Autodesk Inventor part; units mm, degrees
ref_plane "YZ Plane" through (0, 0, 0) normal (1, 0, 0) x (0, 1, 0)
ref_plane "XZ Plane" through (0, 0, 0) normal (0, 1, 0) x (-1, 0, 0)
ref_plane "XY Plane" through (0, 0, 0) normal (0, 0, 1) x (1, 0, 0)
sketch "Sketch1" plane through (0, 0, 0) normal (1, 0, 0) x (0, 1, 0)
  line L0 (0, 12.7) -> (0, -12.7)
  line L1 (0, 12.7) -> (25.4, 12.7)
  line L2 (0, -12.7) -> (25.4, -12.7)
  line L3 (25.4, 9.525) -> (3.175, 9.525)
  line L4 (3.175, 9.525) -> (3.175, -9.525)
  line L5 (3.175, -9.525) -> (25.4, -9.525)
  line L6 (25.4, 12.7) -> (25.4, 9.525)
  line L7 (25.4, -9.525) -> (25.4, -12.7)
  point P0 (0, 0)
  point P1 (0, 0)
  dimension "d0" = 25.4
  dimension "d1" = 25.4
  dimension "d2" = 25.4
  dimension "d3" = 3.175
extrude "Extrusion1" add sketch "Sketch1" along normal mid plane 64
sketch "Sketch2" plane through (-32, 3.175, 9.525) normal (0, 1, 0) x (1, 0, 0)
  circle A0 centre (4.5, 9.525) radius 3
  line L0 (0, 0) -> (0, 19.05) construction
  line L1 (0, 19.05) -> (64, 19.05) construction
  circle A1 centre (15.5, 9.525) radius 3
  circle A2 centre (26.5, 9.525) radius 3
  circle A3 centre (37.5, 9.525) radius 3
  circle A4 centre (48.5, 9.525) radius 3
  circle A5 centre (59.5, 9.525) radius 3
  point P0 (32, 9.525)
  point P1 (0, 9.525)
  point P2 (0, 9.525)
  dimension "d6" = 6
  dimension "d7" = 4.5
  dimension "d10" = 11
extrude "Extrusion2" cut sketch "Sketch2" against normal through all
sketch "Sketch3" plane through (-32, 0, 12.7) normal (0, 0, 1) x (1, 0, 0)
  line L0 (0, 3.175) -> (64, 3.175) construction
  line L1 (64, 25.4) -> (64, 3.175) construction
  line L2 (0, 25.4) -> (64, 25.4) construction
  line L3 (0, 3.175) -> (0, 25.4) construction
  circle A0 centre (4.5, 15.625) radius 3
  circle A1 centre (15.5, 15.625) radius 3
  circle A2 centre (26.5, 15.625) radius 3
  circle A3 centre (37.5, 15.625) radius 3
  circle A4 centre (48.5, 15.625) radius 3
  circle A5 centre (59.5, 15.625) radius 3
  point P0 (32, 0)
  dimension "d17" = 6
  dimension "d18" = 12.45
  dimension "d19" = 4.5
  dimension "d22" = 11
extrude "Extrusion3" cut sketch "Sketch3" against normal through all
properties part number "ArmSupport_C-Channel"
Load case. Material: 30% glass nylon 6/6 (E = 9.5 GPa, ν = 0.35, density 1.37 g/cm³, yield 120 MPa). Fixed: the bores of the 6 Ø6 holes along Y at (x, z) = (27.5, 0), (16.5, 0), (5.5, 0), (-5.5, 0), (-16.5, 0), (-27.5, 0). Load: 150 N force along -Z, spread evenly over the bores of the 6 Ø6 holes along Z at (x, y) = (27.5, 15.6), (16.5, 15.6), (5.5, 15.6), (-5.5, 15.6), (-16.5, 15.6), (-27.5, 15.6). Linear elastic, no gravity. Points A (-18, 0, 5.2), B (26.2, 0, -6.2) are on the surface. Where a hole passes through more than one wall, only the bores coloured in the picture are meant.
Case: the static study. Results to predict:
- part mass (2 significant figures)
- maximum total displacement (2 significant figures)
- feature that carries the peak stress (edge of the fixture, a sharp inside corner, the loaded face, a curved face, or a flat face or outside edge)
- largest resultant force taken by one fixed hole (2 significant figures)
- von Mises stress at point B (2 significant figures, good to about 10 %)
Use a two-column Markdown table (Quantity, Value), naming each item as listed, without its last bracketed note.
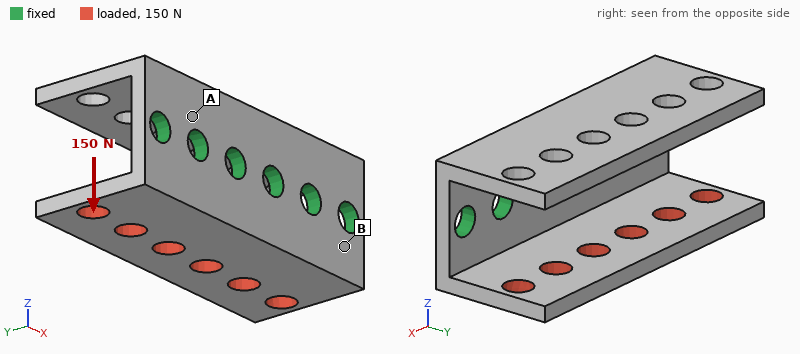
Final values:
| Quantity | Value |
|---|---|
| part mass | 17 g |
| maximum total displacement | 0.39 mm |
| feature that carries the peak stress | a flat face or outside edge |
| largest resultant force taken by one fixed hole | 30 N |
| von Mises stress at point B | 17 MPa |
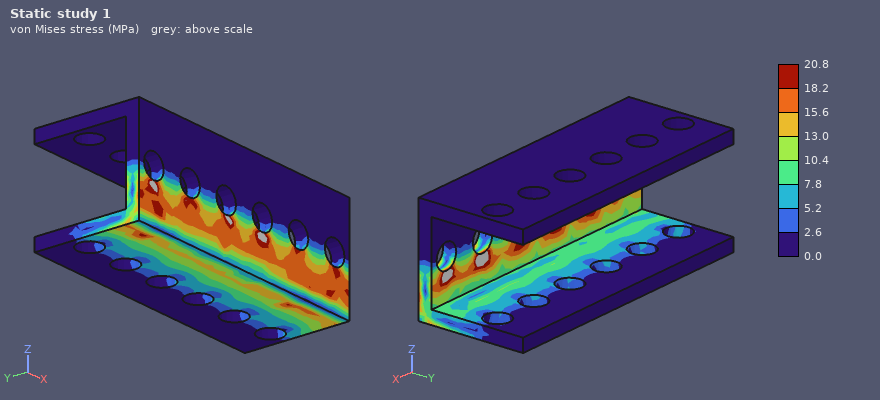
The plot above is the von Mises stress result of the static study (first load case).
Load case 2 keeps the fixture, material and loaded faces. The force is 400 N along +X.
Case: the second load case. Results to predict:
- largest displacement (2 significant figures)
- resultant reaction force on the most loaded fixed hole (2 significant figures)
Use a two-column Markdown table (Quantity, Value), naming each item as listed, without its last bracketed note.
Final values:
| Quantity | Value |
|---|---|
| largest displacement | 0.14 mm |
| resultant reaction force on the most loaded fixed hole | 110 N |
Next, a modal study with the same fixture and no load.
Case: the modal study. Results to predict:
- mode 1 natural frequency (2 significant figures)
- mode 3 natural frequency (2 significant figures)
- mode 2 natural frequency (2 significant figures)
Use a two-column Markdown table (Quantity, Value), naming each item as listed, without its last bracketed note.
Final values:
| Quantity | Value |
|---|---|
| mode 1 natural frequency | 1700 Hz |
| mode 3 natural frequency | 2400 Hz |
| mode 2 natural frequency | 1700 Hz |
